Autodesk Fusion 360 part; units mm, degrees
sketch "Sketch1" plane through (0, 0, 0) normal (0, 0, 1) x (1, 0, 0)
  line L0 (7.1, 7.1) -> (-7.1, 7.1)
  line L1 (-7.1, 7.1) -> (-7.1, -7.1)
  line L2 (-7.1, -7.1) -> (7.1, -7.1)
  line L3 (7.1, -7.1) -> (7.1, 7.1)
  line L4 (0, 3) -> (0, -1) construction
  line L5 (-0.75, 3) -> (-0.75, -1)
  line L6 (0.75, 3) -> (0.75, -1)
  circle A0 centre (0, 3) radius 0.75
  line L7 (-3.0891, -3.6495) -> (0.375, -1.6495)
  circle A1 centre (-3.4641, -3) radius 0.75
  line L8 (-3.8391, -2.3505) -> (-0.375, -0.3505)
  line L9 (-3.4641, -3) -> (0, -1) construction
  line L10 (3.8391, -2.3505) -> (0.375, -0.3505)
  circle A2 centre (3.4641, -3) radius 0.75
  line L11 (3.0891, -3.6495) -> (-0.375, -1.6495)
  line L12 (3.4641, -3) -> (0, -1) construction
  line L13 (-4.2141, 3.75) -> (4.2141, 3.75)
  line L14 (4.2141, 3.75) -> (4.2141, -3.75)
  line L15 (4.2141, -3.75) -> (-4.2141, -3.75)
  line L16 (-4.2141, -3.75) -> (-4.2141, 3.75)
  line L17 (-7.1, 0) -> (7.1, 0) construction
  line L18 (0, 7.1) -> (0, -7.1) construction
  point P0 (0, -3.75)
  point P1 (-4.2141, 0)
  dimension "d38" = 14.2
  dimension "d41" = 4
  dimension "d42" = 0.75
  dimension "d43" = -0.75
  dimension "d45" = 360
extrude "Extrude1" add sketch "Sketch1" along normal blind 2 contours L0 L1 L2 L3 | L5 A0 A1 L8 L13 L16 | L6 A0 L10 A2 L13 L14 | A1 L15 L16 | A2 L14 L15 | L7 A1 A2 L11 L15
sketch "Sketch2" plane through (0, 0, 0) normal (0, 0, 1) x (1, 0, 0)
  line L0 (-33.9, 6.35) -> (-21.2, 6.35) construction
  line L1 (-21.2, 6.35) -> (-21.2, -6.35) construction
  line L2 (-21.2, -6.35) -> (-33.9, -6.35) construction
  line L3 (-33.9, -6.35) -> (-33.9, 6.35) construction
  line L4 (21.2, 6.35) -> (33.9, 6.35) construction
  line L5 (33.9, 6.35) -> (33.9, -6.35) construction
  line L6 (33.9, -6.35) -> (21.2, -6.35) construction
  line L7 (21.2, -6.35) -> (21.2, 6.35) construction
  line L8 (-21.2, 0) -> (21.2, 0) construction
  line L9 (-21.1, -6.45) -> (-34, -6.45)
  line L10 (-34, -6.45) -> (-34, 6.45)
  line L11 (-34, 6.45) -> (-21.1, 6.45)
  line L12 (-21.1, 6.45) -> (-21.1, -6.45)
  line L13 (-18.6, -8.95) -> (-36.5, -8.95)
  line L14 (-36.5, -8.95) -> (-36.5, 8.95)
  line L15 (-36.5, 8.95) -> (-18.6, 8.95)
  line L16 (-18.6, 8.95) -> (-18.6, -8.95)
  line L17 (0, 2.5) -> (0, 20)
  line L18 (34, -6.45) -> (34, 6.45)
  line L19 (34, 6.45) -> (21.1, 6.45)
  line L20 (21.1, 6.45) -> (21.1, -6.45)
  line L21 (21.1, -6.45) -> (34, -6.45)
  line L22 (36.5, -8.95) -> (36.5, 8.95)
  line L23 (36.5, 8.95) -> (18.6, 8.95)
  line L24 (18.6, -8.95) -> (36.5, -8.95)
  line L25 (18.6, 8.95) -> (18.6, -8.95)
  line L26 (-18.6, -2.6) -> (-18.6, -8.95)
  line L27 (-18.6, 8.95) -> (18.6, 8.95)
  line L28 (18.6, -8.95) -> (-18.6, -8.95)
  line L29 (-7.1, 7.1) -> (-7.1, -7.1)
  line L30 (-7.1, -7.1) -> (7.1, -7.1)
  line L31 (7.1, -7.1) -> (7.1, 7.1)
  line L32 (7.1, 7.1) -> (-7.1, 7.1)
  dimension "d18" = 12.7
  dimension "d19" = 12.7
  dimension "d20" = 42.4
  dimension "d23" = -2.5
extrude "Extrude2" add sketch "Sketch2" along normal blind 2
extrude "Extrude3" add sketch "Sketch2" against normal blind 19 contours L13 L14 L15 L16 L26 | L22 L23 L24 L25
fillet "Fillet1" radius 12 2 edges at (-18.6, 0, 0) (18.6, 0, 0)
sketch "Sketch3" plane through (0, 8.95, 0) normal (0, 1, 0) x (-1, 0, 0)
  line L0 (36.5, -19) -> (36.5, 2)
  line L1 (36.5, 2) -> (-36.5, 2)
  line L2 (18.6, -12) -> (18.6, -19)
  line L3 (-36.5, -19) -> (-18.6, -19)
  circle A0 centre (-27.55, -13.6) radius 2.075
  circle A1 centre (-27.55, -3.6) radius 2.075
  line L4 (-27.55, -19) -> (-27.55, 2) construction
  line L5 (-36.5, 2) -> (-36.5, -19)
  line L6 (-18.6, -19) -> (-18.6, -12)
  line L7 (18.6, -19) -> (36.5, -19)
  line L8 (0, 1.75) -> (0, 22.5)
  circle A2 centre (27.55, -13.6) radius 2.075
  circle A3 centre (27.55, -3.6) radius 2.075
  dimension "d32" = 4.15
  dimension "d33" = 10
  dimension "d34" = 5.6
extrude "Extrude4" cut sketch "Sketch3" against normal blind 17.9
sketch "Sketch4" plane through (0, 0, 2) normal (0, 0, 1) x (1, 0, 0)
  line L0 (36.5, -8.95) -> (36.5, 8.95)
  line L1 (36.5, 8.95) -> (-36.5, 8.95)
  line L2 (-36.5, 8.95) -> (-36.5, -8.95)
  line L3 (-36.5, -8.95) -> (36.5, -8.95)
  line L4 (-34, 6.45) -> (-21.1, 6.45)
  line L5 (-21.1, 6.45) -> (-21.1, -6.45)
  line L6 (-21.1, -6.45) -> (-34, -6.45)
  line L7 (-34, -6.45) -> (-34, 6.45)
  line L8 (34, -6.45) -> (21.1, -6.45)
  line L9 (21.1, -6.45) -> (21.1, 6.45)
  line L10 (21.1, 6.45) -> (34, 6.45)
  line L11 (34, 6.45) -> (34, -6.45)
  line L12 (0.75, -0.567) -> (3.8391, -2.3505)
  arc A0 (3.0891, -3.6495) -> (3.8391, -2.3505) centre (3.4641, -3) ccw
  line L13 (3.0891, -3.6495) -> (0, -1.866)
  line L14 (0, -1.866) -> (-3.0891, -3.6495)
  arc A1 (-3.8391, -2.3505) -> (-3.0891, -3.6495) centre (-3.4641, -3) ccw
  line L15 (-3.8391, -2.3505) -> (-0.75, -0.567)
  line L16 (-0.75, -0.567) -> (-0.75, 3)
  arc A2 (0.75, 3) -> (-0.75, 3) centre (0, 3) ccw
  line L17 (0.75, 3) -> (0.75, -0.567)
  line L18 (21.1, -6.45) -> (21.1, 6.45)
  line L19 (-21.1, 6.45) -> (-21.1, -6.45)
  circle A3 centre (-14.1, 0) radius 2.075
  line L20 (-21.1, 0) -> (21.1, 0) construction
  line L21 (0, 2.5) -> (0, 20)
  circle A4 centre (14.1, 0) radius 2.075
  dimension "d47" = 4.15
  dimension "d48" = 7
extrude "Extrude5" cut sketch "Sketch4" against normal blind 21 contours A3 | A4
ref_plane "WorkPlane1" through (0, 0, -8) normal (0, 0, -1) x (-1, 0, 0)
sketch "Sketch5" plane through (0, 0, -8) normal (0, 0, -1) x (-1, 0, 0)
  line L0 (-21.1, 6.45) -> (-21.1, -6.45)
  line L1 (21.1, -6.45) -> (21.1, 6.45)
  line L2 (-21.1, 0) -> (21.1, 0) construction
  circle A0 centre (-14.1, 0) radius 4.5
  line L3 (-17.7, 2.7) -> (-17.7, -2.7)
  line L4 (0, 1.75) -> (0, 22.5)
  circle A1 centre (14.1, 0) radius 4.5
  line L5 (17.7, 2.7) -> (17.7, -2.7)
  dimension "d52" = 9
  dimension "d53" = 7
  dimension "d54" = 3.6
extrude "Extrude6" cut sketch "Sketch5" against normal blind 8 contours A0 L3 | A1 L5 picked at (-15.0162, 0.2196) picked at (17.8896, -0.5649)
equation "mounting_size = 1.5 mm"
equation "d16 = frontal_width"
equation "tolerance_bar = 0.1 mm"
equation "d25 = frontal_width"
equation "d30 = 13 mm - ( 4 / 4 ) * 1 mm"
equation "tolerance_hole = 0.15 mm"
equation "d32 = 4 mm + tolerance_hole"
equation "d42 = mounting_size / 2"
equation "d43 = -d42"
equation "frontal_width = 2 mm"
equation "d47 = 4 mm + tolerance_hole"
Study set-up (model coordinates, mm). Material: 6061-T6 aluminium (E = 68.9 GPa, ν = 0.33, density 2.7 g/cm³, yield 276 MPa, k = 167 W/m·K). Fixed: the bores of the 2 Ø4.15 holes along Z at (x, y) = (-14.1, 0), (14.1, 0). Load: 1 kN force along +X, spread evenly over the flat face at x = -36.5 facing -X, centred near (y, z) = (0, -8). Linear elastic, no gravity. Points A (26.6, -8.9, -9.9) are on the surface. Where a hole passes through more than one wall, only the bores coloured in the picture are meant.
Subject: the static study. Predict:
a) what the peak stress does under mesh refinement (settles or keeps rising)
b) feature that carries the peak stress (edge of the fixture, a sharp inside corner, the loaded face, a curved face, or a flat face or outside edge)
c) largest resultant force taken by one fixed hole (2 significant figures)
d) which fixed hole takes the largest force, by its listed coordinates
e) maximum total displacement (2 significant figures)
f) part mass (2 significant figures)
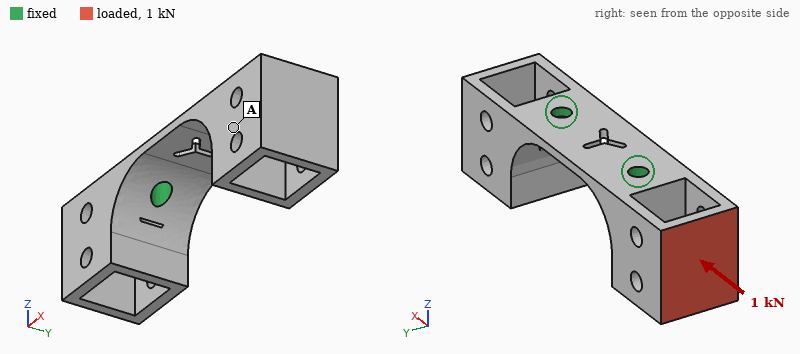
keeps rising
edge of the fixture
1.0 kN
(-14.1, 0)
0.11 mm
22 g
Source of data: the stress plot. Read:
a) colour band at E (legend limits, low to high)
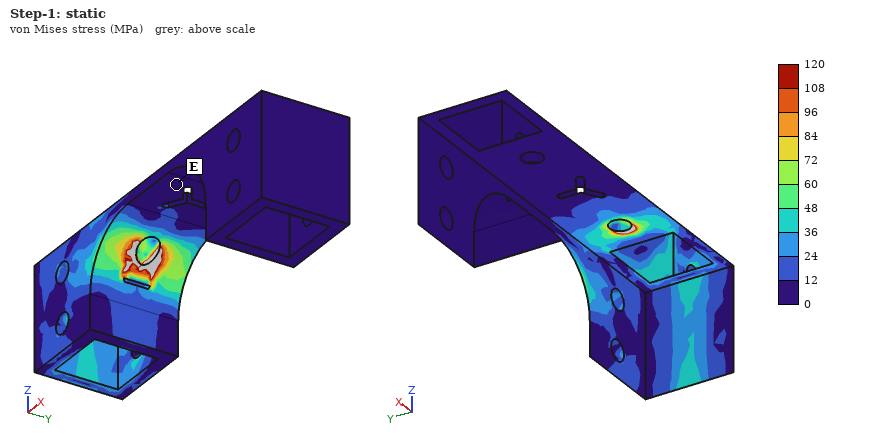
0 to 12 MPa
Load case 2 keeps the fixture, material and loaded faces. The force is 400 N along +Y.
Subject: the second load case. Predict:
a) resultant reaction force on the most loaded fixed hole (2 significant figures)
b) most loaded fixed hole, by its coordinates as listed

530 N
(-14.1, 0)
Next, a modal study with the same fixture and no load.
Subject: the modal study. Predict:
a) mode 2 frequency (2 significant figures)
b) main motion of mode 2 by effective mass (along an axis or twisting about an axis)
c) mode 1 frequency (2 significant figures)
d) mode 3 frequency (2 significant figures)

3700 Hz
along Y
2600 Hz
4800 Hz
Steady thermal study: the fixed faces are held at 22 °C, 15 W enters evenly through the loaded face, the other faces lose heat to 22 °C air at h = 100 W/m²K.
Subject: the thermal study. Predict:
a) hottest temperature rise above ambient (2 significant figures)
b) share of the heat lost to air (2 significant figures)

23 K
23 %
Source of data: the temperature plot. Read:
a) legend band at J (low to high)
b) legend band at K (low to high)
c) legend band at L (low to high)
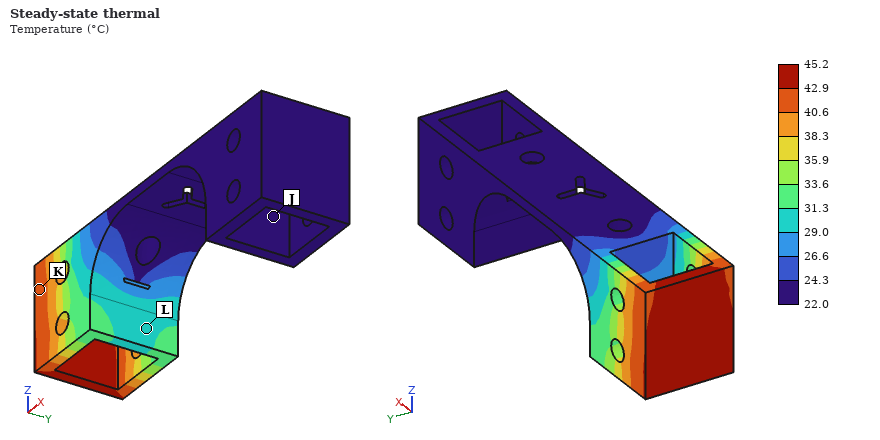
22.0 to 24.3 °C
40.6 to 42.9 °C
29.0 to 31.3 °C
